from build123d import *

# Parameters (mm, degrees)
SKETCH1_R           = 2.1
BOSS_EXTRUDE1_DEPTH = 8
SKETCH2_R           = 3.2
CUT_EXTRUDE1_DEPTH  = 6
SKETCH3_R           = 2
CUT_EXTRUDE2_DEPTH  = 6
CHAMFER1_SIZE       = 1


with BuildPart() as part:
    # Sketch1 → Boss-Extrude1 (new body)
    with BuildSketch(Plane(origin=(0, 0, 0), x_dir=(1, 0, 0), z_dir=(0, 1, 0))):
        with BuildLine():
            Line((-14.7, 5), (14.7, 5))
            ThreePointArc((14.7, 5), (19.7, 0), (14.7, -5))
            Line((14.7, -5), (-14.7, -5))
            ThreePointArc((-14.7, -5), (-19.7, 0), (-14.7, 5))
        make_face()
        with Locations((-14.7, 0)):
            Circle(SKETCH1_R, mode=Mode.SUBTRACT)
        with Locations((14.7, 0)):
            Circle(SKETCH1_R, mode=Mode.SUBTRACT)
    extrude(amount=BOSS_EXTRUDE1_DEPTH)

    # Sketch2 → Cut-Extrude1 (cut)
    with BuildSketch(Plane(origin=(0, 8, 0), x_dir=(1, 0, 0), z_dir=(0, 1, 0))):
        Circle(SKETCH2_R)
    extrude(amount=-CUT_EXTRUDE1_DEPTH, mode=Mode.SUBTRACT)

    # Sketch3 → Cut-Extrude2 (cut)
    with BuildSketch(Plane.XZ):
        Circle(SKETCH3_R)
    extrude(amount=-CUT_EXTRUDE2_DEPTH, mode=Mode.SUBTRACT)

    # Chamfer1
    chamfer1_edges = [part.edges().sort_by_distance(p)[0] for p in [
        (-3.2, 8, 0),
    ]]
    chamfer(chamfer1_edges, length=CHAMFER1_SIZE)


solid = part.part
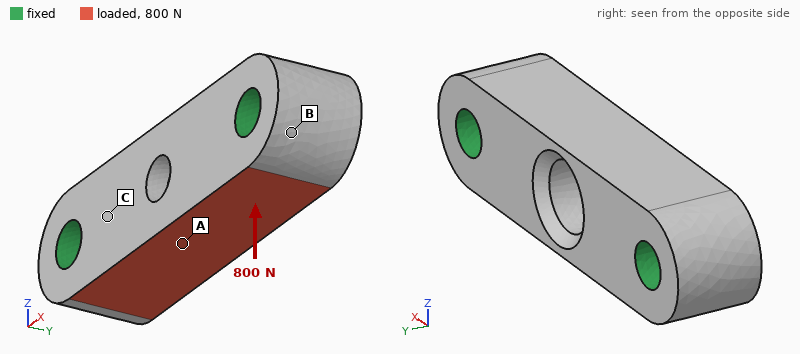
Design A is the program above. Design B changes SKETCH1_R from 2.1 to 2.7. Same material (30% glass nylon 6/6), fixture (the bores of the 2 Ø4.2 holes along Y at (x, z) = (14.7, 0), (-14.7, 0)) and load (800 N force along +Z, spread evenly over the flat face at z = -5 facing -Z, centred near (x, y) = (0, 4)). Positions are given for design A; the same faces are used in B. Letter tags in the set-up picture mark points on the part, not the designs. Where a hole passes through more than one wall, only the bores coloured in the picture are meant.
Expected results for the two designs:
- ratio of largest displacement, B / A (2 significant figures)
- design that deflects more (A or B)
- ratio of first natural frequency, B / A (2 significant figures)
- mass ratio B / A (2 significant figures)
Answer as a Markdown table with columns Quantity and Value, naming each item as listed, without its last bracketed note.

| Quantity | Value |
|---|---|
| ratio of largest displacement, B / A | 0.86 |
| design that deflects more | A |
| ratio of first natural frequency, B / A | 1.1 |
| mass ratio B / A | 0.94 |
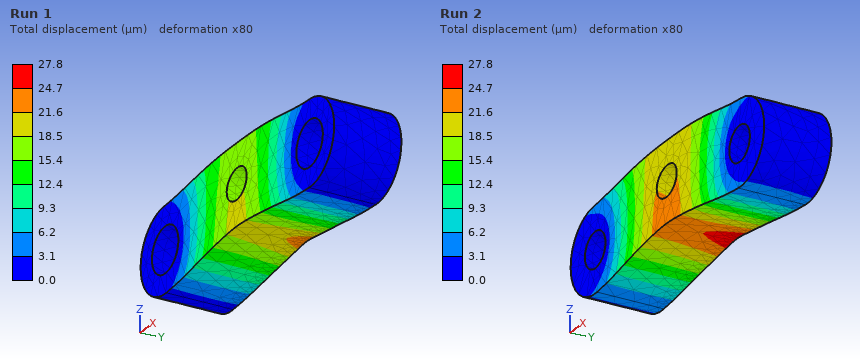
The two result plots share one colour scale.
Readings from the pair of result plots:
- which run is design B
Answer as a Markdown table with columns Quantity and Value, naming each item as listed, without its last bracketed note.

| Quantity | Value |
|---|---|
| which run is design B | Run 1 |
